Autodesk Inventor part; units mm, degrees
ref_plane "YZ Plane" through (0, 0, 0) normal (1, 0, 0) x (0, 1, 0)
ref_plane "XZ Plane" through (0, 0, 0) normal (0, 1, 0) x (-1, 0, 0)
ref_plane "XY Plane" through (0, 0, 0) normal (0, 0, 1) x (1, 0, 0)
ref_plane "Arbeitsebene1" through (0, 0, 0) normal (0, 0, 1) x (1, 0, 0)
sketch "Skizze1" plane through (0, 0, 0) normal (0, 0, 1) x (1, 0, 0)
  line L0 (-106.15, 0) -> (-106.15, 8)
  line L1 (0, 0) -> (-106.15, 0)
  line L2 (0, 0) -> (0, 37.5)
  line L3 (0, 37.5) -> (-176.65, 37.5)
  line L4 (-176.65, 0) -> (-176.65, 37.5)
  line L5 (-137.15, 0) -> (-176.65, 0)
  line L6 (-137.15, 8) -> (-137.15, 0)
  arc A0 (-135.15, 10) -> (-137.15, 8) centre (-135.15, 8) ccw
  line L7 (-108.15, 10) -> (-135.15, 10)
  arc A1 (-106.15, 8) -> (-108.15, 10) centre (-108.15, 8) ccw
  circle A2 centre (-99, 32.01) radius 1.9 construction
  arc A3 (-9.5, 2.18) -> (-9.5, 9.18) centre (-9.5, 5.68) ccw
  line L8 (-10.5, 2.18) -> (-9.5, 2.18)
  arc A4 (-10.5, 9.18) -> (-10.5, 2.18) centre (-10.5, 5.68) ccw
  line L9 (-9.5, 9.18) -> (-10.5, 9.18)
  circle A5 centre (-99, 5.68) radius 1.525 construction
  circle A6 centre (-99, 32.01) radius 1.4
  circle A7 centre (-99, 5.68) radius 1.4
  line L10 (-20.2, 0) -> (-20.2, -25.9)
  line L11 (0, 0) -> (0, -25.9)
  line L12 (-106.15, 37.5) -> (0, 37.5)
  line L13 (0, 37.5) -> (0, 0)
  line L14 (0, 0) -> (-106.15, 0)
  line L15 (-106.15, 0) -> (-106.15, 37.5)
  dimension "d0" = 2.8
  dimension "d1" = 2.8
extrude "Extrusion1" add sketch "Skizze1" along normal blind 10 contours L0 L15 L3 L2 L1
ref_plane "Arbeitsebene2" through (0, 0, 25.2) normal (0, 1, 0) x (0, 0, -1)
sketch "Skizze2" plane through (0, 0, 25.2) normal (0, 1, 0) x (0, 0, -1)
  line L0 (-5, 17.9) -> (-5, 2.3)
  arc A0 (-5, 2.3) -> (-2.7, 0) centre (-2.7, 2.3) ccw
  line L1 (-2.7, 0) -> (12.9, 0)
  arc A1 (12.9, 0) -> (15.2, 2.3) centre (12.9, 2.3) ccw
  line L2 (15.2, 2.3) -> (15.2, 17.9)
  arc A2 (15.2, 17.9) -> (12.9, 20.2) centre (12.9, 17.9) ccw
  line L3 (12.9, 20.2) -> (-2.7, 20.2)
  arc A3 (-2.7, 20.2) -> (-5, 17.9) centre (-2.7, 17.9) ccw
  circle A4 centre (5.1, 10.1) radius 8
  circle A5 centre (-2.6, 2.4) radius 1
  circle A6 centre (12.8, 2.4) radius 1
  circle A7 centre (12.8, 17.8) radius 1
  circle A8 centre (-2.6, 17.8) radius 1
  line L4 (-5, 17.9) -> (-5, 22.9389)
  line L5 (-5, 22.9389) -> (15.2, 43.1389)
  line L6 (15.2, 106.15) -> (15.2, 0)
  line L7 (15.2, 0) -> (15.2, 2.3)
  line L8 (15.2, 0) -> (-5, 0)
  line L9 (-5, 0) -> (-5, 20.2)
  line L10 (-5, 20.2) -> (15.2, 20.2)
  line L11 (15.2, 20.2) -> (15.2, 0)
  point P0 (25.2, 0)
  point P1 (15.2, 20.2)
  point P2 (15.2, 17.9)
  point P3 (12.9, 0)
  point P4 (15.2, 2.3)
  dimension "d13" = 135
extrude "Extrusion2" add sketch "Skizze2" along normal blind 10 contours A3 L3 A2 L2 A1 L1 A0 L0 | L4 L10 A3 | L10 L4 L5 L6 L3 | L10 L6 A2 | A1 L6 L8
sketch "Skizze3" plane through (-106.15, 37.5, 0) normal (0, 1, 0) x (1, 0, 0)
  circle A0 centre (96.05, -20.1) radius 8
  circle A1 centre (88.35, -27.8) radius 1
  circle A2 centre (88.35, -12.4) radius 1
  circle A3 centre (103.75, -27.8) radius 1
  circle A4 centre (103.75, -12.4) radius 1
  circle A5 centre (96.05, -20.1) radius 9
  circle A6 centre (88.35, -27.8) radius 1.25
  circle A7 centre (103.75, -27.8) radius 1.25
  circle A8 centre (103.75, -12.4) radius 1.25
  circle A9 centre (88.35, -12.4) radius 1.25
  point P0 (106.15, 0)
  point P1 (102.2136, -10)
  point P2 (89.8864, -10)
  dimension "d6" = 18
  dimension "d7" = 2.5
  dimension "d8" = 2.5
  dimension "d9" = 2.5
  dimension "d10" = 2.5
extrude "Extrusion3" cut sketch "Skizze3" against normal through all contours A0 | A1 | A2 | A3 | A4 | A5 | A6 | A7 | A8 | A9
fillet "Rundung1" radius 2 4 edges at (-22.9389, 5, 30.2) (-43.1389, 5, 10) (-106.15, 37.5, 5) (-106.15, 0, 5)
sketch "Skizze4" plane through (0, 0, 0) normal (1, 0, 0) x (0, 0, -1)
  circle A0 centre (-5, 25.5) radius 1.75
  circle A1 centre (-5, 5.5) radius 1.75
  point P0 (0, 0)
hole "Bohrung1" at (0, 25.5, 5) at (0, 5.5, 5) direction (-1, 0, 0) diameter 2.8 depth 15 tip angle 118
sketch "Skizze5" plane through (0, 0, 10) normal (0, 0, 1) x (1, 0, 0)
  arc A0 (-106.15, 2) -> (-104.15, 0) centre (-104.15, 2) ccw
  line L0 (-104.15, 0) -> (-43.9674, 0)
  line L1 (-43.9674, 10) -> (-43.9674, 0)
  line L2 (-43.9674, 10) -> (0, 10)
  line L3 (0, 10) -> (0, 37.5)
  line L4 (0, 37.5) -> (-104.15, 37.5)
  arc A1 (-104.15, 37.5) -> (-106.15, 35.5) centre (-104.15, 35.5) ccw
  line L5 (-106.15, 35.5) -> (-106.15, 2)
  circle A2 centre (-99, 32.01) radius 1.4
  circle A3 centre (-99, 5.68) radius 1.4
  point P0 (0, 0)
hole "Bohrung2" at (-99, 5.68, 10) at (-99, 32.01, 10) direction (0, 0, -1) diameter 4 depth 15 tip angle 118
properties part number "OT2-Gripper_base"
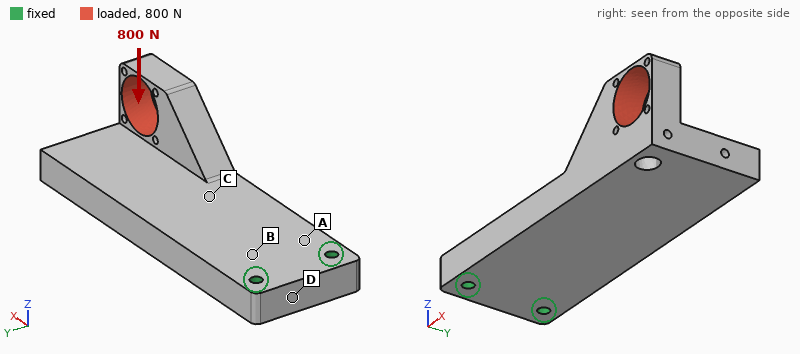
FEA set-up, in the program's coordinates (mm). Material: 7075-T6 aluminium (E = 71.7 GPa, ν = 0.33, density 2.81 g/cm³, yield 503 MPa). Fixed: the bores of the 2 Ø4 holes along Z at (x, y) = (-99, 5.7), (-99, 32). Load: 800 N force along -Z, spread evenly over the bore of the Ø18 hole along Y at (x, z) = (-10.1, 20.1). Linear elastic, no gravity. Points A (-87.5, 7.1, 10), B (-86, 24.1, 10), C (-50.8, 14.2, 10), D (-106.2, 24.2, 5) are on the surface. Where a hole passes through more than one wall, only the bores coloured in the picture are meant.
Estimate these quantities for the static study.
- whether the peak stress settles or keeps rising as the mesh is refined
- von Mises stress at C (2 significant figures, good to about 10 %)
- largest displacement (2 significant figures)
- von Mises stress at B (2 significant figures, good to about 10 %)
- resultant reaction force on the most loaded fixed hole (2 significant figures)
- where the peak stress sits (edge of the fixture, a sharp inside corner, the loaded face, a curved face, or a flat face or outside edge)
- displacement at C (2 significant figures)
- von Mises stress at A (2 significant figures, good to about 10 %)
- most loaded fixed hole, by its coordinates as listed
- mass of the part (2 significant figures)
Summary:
keeps rising
56 MPa
1.1 mm
89 MPa
770 N
edge of the fixture
0.35 mm
110 MPa
(-99, 5.7)
120 g
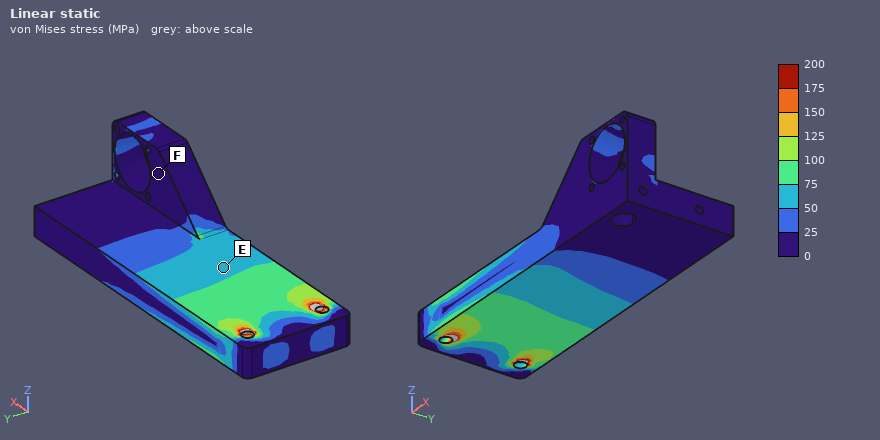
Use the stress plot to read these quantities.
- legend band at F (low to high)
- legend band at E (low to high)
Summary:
0 to 25 MPa
50 to 75 MPa
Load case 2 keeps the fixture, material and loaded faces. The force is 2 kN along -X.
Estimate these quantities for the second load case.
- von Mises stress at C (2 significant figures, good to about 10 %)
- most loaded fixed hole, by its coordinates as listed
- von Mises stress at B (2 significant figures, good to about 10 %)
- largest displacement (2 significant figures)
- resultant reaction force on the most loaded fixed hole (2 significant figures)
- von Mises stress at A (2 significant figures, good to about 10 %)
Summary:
57 MPa
(-99, 5.7)
46 MPa
0.69 mm
2.0 kN
64 MPa
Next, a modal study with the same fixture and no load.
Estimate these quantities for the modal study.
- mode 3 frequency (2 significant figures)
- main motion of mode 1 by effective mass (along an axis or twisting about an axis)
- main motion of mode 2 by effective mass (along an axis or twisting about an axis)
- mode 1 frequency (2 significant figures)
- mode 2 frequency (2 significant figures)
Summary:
3400 Hz
along Z
along Y
740 Hz
2500 Hz
